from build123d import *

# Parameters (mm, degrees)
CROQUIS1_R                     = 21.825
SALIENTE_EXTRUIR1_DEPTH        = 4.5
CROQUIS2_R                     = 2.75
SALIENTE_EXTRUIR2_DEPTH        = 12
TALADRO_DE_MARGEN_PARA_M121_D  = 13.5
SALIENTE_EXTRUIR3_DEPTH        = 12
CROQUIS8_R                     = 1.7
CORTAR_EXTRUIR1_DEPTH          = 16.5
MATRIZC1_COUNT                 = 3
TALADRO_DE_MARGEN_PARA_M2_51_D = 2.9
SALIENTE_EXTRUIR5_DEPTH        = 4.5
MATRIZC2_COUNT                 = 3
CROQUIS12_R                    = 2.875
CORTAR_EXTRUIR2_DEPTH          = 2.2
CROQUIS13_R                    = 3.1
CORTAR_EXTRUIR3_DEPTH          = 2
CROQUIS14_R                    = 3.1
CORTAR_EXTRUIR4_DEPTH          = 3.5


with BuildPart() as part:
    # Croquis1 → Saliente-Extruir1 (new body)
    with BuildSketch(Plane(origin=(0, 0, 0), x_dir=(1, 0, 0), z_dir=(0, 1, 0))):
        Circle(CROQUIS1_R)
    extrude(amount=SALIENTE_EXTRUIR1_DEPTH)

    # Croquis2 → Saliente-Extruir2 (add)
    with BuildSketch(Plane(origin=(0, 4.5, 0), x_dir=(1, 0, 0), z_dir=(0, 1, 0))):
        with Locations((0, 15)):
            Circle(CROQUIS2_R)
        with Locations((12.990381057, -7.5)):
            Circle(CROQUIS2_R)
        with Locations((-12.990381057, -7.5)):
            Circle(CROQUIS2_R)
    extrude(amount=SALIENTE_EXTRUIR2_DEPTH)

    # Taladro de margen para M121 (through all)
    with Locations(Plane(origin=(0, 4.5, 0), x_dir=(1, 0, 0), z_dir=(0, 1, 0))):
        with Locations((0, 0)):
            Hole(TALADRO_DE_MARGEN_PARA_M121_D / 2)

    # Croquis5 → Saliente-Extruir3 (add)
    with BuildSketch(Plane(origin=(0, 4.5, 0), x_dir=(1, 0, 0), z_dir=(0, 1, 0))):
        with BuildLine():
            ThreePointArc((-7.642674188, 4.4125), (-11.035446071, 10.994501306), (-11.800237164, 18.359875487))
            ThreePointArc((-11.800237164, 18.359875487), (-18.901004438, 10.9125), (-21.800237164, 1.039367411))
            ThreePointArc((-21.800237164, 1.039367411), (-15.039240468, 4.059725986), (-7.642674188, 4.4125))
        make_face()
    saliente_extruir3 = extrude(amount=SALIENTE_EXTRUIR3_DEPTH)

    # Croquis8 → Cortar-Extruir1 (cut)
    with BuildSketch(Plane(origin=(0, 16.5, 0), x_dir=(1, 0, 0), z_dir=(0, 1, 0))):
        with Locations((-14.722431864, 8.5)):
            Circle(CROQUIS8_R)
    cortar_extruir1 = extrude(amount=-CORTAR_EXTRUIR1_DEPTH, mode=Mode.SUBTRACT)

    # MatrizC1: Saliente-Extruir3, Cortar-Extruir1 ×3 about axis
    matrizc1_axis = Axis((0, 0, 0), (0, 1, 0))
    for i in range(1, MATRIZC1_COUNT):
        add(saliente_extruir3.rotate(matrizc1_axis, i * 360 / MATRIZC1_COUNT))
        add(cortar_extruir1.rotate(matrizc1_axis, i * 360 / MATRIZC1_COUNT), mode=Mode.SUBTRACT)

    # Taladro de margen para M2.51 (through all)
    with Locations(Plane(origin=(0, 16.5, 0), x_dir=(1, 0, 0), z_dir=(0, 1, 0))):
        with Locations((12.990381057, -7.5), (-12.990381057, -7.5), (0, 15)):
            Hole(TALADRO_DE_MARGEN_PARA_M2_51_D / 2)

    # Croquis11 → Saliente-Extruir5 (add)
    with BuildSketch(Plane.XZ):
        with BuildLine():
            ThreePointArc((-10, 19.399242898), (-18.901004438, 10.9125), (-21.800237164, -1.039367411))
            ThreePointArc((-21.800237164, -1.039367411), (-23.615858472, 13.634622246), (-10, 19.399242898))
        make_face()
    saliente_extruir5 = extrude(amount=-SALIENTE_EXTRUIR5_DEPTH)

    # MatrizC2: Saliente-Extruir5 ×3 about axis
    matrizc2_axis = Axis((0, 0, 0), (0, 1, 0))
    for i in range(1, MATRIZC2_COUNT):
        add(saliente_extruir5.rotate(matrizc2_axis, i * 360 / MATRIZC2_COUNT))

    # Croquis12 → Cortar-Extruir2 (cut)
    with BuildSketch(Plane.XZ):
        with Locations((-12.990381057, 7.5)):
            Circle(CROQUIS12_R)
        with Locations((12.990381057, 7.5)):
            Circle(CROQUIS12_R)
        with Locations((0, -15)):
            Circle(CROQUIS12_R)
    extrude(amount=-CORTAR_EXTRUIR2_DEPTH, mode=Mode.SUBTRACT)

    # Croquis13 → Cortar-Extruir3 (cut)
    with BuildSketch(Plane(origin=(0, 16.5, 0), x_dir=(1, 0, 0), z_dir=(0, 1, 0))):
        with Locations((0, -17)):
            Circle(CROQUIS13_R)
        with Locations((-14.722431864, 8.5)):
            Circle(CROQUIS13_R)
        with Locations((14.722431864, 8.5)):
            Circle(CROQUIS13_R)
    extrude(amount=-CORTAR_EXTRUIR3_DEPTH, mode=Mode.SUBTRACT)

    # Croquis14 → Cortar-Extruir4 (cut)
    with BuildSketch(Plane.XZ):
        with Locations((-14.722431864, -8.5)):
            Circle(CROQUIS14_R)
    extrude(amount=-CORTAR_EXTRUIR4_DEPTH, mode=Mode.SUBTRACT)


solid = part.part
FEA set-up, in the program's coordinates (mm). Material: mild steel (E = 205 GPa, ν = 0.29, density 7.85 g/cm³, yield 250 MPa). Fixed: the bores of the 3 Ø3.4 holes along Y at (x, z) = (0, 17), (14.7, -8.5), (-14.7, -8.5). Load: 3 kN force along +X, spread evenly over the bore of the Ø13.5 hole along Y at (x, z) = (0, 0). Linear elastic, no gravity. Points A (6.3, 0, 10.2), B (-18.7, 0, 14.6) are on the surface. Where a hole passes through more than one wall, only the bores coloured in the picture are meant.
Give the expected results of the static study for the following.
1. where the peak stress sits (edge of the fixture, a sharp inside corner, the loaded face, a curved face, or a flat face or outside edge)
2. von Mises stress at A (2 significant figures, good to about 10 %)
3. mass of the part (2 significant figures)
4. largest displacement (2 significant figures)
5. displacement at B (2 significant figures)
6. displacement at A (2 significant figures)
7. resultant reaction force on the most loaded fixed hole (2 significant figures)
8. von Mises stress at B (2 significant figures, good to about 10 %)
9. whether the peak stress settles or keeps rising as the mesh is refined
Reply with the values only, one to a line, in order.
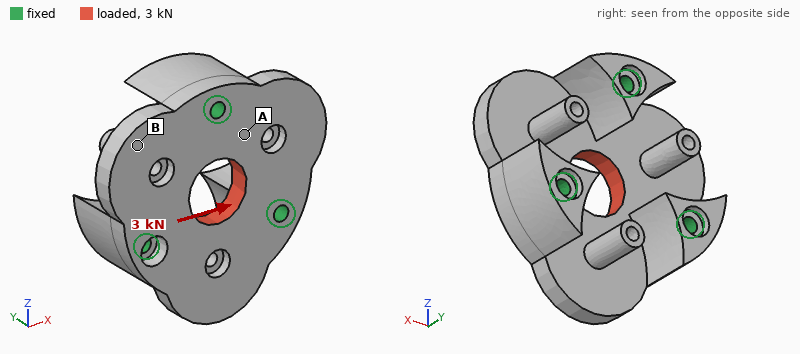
edge of the fixture
12 MPa
88 g
2.1 µm
1.2 µm
1.1 µm
1.1 kN
5.3 MPa
keeps rising
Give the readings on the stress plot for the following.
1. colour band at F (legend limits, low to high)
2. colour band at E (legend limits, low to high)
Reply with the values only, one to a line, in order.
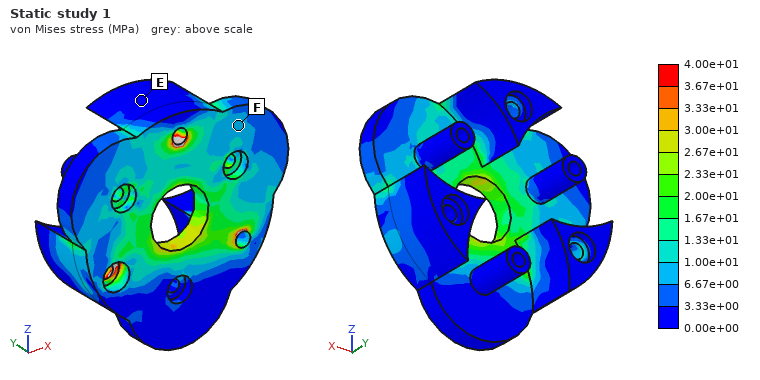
6.67e+00 to 1.00e+01 MPa
0.00e+00 to 3.33e+00 MPa
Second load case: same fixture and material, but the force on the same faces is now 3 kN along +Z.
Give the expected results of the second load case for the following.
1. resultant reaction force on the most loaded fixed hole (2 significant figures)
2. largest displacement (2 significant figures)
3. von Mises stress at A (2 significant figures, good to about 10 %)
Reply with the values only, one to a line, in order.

1.1 kN
2.4 µm
11 MPa
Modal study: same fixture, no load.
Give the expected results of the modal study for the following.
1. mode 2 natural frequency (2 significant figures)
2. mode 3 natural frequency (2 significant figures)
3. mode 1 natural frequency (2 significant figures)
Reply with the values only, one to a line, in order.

14 kHz
14 kHz
13 kHz
